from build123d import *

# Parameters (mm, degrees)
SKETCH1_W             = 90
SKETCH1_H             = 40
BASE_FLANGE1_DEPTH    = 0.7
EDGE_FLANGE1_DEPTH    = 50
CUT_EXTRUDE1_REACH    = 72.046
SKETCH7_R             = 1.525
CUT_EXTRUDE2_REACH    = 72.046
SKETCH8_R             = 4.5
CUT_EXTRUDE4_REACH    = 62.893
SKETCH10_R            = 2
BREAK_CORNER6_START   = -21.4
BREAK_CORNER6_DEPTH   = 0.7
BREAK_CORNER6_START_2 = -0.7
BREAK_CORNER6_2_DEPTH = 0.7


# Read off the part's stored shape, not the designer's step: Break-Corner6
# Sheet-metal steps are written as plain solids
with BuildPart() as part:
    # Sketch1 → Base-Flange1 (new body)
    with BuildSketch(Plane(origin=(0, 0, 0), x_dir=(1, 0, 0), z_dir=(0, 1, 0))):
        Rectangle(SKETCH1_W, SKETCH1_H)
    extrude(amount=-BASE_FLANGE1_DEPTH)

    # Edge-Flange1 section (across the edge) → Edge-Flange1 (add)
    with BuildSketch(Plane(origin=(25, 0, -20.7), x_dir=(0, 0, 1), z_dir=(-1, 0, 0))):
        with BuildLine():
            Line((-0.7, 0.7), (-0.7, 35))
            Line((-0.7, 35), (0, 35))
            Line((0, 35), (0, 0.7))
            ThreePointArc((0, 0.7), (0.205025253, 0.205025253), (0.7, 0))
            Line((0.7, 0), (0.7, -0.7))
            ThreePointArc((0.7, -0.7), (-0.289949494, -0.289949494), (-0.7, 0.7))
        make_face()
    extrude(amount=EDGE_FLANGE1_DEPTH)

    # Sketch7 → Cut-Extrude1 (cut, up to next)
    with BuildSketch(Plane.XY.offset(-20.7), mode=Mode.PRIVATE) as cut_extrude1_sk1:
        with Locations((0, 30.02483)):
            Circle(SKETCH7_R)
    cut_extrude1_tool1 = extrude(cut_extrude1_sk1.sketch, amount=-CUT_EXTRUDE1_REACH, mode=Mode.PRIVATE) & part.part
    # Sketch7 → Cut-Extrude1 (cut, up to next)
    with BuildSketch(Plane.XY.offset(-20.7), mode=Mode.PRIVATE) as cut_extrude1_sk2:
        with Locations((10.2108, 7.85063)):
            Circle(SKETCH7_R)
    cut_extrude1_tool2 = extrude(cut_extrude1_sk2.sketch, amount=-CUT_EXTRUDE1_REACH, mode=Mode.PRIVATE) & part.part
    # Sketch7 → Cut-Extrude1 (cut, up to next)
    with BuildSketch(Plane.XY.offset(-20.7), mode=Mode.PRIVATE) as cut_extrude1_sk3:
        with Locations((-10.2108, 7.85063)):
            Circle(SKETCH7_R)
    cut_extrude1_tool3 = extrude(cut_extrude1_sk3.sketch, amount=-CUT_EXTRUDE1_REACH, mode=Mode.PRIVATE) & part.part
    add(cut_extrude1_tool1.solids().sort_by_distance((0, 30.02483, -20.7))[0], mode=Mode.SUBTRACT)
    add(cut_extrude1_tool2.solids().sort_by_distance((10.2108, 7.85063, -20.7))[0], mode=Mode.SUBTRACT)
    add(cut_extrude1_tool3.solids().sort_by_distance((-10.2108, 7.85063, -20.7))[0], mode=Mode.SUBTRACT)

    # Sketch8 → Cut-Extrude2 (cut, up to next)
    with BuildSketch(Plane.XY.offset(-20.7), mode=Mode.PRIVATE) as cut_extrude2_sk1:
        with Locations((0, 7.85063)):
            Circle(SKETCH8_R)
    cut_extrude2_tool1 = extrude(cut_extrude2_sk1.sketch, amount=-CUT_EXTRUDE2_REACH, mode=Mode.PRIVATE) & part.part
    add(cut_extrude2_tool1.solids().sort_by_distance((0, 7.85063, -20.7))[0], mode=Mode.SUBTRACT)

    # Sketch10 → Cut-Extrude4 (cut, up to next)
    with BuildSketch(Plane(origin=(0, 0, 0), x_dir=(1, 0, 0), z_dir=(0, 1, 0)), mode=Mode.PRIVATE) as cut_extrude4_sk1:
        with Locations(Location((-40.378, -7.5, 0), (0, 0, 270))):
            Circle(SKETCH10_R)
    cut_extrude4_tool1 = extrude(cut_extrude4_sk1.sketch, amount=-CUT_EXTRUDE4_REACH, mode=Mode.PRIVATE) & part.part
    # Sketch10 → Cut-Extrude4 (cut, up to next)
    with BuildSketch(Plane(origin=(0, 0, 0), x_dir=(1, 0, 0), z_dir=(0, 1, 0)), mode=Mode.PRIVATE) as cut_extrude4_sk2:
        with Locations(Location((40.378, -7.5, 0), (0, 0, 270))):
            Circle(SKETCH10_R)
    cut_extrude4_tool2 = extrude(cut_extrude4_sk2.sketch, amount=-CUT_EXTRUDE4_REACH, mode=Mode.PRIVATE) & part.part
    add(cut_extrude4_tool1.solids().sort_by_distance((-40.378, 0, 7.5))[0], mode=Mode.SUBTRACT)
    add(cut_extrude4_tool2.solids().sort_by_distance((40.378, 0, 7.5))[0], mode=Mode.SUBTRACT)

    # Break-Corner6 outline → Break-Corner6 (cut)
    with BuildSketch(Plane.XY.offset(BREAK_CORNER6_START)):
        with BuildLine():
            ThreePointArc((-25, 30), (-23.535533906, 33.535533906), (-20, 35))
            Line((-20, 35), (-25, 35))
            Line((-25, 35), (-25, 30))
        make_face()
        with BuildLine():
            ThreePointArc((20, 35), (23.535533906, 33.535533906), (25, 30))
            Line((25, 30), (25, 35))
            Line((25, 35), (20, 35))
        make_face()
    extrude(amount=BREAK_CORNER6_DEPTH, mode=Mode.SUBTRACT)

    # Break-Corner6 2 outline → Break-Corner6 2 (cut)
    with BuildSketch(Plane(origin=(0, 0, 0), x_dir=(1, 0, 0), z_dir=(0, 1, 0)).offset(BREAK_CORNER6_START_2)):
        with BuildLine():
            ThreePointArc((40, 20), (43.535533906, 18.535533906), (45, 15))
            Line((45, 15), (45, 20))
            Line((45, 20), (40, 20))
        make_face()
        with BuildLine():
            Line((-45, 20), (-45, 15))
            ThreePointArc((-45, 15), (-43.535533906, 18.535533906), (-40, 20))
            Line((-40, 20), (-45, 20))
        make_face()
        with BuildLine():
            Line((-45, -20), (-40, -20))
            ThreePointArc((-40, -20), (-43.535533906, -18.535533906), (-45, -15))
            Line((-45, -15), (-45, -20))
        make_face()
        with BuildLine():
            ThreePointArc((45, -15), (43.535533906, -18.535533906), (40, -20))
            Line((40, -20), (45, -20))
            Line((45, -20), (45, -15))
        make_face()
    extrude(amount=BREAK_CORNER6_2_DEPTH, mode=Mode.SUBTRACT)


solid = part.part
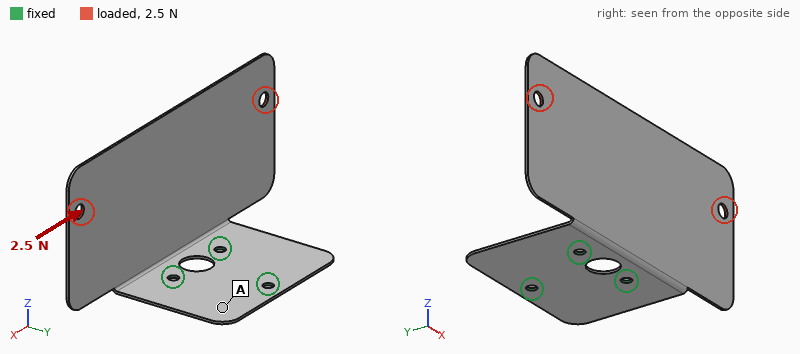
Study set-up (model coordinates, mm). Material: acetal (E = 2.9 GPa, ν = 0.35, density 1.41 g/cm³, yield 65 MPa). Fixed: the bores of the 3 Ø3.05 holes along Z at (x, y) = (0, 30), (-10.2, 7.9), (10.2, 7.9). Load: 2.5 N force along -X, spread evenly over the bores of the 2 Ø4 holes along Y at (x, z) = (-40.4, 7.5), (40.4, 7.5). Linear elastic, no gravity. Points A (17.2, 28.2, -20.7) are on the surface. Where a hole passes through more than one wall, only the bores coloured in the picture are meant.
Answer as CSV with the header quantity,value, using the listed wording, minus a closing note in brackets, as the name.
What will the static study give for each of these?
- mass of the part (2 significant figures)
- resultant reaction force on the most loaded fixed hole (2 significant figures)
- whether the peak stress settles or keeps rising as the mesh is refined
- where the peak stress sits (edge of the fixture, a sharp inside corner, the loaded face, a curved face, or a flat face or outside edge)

quantity,value
mass of the part,5.2 g
resultant reaction force on the most loaded fixed hole,3.3 N
whether the peak stress settles or keeps rising as the mesh is refined,keeps rising
where the peak stress sits,edge of the fixture
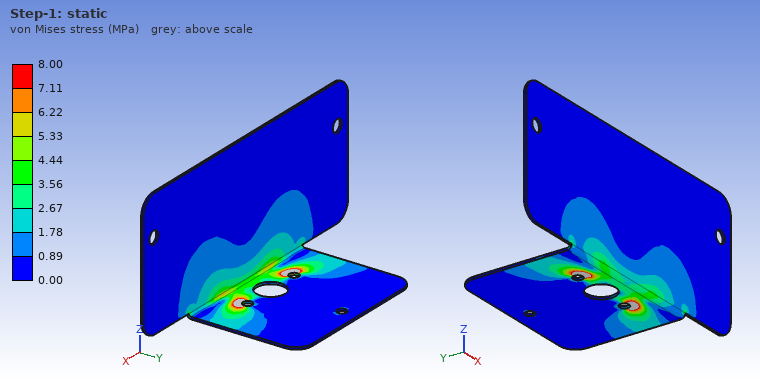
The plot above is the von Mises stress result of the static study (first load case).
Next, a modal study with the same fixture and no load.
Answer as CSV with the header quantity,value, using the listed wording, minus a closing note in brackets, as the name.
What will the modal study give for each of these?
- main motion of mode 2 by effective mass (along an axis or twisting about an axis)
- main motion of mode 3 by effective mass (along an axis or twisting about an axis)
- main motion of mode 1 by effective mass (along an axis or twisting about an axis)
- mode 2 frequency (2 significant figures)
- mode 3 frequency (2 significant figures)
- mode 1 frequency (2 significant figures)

quantity,value
main motion of mode 2 by effective mass,twisting about Z
main motion of mode 3 by effective mass,along X
main motion of mode 1 by effective mass,along Y
mode 2 frequency,85 Hz
mode 3 frequency,170 Hz
mode 1 frequency,57 Hz
